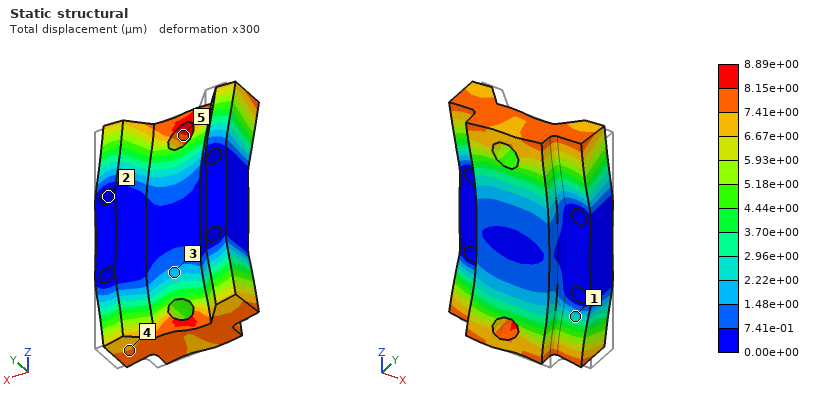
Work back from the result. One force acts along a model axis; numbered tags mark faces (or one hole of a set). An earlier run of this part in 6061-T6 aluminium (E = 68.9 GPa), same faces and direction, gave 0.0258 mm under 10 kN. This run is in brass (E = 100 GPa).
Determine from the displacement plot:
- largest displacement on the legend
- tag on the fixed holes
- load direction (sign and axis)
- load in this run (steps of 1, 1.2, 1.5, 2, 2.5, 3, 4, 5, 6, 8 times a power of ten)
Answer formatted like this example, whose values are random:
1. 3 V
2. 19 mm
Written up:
1. 8.89e+00 µm
2. 2
3. -X
4. 5 kN
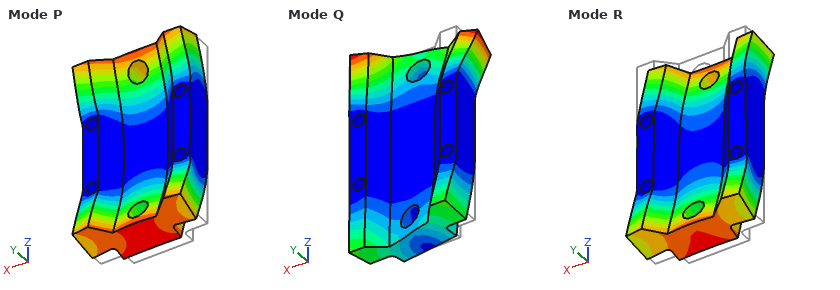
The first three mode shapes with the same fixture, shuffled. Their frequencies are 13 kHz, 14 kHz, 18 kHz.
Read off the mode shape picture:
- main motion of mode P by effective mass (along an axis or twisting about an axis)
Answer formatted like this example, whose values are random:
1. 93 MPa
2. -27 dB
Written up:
1. along Y
